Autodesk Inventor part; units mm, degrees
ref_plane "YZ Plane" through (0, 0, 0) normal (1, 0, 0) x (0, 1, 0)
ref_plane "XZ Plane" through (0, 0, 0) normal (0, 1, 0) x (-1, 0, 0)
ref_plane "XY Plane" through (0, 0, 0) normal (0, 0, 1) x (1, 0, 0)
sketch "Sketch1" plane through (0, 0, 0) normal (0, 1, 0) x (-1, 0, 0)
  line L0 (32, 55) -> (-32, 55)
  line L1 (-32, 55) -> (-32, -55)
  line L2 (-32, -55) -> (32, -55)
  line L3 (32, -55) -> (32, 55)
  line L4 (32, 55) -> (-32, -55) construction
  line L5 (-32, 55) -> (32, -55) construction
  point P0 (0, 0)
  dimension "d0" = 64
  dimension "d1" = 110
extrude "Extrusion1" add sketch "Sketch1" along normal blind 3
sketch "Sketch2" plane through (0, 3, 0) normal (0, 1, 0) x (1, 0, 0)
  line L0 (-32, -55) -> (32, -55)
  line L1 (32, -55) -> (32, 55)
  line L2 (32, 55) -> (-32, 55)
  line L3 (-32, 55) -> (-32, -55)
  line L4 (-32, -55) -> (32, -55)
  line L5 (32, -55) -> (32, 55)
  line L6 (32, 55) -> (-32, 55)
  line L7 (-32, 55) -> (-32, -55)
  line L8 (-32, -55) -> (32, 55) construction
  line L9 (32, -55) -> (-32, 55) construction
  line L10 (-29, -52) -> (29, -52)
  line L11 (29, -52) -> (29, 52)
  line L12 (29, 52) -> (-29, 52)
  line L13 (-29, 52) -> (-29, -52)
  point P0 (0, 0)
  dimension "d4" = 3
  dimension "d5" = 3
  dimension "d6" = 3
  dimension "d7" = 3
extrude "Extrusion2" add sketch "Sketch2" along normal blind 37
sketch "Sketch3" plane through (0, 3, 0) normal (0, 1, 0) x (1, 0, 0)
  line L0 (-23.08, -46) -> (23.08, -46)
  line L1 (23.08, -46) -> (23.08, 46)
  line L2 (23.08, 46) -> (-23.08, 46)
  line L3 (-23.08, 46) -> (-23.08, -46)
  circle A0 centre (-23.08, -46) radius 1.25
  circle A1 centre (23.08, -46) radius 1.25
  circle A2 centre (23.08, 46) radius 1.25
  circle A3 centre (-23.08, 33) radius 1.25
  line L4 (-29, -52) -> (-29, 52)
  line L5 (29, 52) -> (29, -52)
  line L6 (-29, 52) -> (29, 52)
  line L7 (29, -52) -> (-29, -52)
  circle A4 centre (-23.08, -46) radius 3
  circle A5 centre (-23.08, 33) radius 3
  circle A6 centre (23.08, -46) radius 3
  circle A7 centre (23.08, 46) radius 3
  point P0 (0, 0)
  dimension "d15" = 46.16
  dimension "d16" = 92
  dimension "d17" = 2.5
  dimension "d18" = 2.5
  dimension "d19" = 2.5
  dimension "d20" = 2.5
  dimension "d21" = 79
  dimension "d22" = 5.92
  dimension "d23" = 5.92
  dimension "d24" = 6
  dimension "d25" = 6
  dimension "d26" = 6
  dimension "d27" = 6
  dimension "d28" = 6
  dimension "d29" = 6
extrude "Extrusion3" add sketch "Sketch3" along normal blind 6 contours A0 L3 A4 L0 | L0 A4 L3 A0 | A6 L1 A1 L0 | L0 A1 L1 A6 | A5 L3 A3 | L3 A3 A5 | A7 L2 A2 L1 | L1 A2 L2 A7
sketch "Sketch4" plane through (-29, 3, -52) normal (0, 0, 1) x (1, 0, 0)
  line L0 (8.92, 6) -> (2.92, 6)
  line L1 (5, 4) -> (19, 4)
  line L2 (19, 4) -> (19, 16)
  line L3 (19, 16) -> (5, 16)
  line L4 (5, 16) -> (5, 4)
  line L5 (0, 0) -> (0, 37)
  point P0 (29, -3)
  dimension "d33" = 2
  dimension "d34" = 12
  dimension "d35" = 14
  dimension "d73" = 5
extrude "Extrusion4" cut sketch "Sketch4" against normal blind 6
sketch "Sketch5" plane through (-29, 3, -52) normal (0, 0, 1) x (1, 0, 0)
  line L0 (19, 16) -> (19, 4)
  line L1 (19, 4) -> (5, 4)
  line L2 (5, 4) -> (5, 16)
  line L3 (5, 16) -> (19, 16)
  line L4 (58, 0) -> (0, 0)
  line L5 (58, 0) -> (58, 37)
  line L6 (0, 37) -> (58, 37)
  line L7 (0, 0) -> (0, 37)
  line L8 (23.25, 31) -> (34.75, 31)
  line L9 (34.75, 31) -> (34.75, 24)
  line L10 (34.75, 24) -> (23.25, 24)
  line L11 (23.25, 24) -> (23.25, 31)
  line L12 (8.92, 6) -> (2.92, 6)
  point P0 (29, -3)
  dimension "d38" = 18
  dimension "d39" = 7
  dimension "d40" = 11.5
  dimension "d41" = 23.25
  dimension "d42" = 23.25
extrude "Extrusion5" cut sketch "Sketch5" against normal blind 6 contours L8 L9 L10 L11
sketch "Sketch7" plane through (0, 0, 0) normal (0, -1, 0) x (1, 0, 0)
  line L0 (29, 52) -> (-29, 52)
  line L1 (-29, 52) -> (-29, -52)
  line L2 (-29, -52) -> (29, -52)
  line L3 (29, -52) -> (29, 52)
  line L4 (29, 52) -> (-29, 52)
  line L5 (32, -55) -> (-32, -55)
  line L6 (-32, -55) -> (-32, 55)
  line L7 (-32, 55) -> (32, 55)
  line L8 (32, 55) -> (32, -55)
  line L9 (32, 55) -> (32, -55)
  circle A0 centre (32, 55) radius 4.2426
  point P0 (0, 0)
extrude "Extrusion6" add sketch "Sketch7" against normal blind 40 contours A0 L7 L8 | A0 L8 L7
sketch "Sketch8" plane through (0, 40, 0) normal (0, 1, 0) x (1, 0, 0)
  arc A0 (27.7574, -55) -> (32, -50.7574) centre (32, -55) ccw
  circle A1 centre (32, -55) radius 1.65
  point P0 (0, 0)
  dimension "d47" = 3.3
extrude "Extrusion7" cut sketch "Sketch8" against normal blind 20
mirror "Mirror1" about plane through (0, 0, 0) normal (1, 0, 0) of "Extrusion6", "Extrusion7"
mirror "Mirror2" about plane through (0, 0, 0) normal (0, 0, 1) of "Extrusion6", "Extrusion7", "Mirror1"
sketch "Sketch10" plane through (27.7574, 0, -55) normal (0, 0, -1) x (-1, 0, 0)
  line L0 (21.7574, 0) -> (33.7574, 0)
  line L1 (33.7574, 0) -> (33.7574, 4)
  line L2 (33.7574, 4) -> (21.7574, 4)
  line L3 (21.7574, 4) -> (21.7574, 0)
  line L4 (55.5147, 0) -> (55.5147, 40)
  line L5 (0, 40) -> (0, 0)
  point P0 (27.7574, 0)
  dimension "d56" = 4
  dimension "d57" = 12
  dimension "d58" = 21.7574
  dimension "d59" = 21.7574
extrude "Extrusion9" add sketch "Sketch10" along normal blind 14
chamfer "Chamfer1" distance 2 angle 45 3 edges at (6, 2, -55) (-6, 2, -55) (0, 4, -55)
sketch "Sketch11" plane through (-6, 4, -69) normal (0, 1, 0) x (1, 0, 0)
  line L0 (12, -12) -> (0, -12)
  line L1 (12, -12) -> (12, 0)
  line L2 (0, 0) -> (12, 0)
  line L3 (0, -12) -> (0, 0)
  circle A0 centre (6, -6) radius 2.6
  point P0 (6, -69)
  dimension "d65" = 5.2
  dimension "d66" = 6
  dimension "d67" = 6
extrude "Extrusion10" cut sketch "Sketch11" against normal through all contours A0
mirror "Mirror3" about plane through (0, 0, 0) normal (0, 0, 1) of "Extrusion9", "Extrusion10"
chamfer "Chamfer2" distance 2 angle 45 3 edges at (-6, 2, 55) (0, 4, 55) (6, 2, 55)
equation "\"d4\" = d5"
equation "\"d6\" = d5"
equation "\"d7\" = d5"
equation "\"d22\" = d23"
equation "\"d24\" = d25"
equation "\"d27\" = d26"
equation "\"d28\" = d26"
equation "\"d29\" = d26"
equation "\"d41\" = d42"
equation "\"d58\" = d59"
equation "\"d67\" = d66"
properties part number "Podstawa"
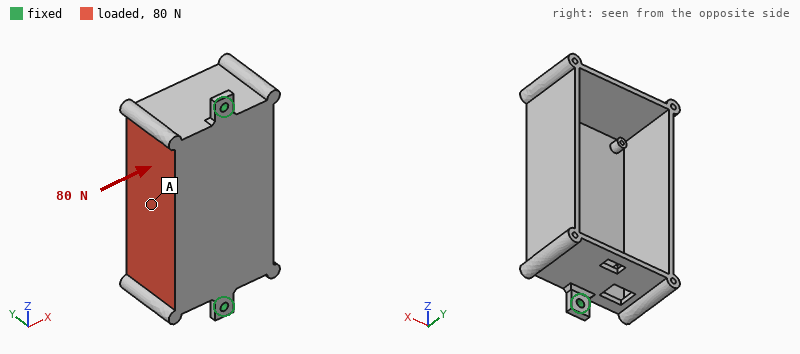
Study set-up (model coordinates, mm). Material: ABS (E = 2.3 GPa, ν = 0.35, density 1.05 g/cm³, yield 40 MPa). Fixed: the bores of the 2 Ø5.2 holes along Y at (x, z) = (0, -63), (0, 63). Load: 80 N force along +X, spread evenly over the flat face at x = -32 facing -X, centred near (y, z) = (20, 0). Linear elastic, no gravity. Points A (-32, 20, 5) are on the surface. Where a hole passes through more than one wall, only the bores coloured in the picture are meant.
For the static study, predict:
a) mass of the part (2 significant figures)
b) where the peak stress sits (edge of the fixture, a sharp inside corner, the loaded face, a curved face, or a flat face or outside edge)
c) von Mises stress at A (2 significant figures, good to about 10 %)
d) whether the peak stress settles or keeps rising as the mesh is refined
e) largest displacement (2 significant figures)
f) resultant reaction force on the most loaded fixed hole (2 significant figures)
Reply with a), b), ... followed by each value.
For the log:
a) 69 g
b) edge of the fixture
c) 1.3 MPa
d) keeps rising
e) 1.7 mm
f) 40 N
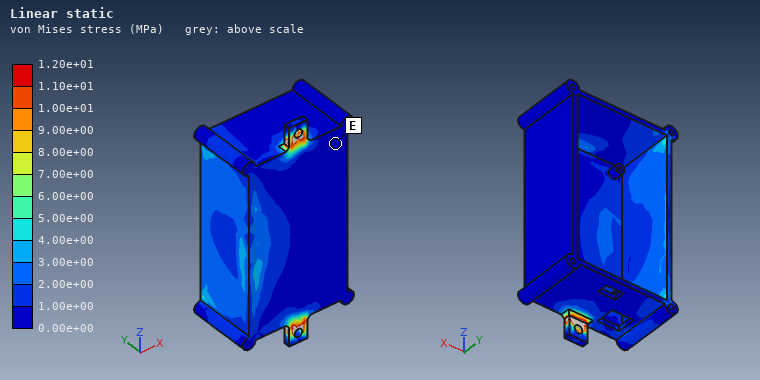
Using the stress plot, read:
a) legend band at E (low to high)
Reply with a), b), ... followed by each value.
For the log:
a) 0.00e+00 to 1.00e+00 MPa
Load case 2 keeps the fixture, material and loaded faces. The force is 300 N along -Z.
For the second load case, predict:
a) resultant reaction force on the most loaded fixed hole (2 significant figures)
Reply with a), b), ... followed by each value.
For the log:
a) 180 N
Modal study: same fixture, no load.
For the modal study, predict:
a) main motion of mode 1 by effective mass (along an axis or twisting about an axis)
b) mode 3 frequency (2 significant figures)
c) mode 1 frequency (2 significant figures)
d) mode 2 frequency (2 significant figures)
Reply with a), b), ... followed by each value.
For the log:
a) along X
b) 570 Hz
c) 170 Hz
d) 310 Hz
